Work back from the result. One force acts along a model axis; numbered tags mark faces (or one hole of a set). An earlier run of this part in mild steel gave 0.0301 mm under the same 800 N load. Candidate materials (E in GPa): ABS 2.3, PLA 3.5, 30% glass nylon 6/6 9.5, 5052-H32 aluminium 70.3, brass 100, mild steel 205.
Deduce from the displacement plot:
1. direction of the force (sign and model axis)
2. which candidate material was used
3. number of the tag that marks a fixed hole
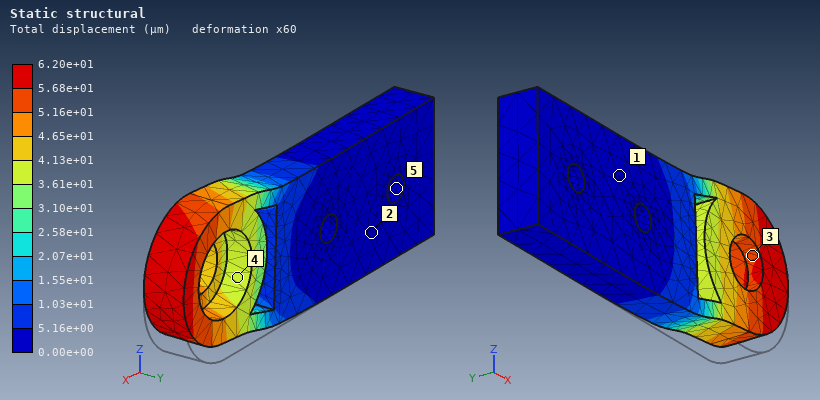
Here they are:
+Z
brass
5
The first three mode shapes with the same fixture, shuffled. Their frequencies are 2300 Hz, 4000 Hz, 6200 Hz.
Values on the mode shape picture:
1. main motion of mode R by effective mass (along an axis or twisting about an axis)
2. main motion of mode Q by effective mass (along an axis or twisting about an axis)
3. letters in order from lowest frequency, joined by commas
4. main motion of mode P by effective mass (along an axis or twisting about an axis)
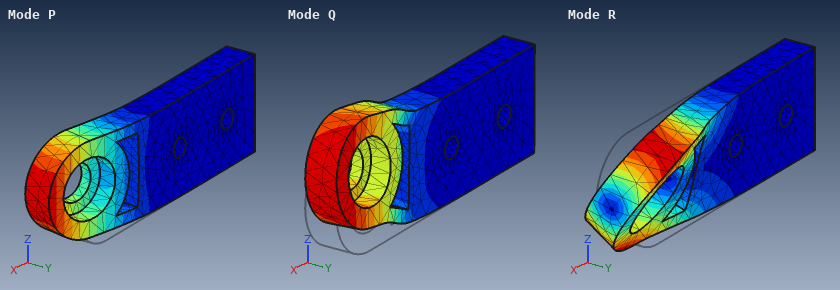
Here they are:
twisting about X
along Z
P, Q, R
along Y
